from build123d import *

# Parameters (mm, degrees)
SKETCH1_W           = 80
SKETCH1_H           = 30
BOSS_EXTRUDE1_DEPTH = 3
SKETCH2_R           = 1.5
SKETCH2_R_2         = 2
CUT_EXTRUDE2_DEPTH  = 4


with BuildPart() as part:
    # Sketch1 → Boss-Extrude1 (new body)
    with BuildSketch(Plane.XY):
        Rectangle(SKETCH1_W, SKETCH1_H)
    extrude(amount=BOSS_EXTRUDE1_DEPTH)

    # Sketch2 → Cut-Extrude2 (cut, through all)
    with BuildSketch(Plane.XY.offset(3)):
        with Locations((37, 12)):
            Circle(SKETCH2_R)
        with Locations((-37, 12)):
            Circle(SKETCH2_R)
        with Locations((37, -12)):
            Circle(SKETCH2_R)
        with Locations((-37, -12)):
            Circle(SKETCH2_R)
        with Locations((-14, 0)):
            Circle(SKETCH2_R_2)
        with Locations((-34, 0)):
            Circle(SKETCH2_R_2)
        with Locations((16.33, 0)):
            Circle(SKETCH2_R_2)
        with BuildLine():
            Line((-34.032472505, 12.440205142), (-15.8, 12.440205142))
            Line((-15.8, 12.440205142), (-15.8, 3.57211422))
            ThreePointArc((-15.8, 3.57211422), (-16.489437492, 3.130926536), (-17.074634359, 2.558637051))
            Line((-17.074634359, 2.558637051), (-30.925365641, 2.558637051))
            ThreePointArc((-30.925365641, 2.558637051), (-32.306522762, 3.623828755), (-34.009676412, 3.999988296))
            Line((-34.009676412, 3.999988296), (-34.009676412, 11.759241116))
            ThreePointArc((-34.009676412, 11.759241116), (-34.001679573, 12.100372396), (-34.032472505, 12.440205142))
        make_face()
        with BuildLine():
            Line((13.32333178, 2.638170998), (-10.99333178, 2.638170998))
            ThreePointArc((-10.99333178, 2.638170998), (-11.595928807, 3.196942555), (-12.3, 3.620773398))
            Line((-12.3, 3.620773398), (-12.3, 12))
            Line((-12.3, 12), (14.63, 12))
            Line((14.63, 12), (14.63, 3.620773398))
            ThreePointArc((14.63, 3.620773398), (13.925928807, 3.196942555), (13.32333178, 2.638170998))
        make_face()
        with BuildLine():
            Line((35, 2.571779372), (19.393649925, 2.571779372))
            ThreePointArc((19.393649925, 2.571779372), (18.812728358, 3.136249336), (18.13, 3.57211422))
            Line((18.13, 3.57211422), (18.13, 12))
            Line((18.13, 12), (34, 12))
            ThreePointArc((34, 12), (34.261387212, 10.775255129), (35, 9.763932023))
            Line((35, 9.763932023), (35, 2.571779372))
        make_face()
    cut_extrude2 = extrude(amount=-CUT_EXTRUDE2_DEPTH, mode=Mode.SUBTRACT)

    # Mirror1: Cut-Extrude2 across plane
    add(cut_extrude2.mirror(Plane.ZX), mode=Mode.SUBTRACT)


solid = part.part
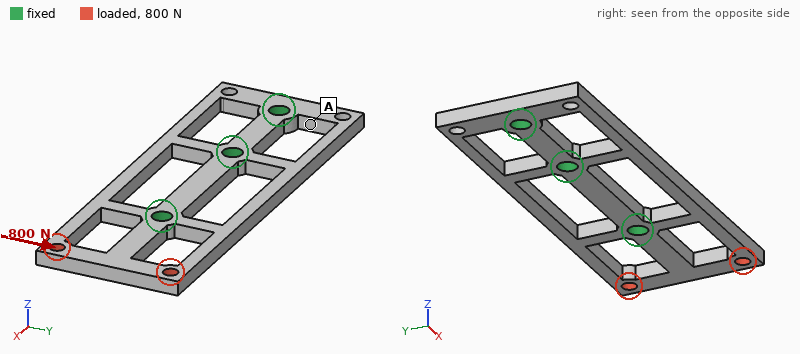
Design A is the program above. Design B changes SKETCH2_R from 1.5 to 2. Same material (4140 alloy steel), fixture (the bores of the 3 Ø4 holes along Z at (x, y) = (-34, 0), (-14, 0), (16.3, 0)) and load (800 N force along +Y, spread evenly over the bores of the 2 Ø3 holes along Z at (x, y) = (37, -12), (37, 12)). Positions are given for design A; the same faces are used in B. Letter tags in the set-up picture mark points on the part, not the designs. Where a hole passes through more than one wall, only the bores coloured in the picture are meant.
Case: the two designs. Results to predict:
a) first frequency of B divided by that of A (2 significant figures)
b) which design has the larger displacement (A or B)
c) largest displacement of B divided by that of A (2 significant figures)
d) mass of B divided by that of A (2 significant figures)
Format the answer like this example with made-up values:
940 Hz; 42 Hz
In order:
1.0; B; 1.1; 0.98
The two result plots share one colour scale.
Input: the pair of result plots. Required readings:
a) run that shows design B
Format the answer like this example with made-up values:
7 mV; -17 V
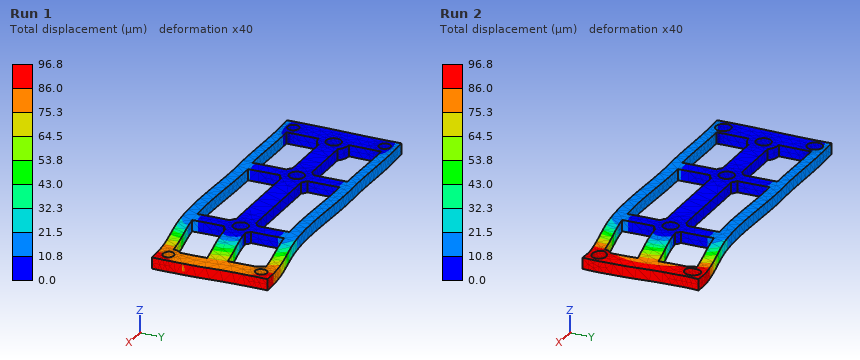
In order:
Run 2
